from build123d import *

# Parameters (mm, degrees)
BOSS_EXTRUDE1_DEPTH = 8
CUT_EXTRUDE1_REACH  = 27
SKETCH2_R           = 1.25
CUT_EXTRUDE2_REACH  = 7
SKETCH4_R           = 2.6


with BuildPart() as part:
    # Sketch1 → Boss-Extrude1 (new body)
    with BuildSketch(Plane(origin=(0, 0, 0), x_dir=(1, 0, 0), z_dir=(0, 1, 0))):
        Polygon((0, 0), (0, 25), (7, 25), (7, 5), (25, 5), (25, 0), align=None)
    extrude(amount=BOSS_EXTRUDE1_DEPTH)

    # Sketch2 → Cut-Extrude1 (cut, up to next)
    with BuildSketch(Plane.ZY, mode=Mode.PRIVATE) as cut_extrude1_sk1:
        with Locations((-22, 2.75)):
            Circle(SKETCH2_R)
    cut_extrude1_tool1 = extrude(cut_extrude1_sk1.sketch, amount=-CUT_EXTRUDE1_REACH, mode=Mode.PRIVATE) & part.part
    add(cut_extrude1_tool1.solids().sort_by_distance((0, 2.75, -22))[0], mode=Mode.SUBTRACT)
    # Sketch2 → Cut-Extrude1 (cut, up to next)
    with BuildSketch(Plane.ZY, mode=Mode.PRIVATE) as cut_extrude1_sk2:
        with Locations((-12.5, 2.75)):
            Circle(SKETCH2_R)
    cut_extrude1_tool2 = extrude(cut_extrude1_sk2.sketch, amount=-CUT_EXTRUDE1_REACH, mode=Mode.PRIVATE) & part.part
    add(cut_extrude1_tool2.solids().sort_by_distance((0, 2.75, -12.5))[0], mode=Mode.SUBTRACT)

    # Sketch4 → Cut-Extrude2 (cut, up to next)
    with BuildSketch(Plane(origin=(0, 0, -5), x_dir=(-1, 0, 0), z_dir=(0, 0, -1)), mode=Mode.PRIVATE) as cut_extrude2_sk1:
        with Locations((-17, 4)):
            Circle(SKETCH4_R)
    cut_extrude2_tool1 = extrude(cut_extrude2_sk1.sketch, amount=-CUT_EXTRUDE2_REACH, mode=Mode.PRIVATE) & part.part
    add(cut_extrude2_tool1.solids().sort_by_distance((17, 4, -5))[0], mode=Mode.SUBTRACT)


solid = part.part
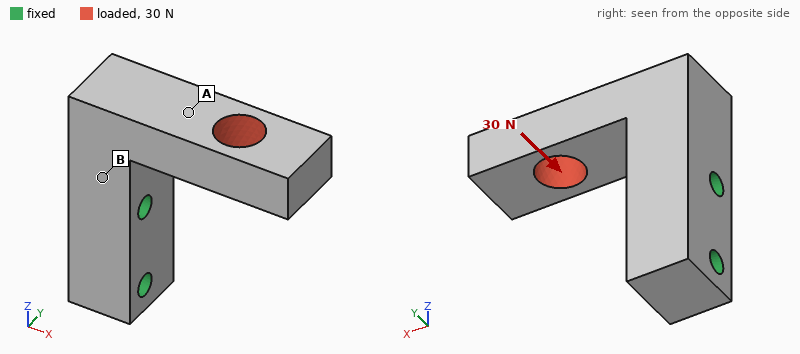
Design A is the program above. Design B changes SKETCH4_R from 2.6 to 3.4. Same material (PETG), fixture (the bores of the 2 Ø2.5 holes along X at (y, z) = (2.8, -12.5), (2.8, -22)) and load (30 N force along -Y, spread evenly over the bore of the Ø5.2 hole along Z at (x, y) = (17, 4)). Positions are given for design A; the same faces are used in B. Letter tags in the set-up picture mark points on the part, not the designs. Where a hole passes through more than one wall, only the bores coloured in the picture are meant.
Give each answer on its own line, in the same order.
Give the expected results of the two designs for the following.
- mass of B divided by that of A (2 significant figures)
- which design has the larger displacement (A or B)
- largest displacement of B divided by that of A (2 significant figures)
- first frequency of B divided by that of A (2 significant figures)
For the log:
0.96
B
1.3
0.97
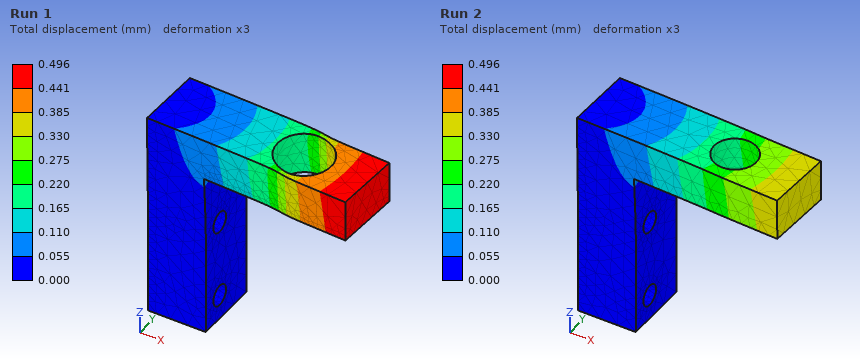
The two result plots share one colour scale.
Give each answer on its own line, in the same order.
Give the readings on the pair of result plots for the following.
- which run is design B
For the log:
Run 1
